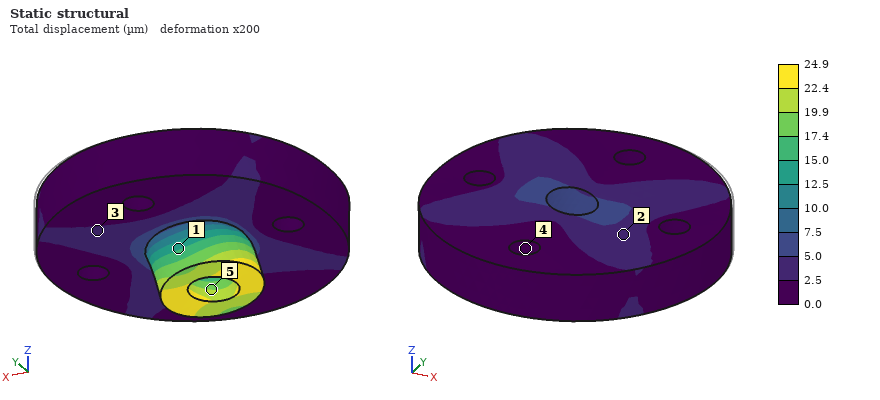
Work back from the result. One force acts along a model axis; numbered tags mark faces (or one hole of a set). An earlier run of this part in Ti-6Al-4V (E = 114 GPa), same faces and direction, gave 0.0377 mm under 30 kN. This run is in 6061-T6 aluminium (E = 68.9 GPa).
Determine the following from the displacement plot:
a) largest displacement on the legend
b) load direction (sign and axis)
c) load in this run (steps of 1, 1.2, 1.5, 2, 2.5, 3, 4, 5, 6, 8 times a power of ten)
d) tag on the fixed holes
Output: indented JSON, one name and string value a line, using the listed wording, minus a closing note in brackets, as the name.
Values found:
{
  "largest displacement on the legend": "24.9 µm",
  "load direction": "-X",
  "load in this run": "12 kN",
  "tag on the fixed holes": "4"
}
